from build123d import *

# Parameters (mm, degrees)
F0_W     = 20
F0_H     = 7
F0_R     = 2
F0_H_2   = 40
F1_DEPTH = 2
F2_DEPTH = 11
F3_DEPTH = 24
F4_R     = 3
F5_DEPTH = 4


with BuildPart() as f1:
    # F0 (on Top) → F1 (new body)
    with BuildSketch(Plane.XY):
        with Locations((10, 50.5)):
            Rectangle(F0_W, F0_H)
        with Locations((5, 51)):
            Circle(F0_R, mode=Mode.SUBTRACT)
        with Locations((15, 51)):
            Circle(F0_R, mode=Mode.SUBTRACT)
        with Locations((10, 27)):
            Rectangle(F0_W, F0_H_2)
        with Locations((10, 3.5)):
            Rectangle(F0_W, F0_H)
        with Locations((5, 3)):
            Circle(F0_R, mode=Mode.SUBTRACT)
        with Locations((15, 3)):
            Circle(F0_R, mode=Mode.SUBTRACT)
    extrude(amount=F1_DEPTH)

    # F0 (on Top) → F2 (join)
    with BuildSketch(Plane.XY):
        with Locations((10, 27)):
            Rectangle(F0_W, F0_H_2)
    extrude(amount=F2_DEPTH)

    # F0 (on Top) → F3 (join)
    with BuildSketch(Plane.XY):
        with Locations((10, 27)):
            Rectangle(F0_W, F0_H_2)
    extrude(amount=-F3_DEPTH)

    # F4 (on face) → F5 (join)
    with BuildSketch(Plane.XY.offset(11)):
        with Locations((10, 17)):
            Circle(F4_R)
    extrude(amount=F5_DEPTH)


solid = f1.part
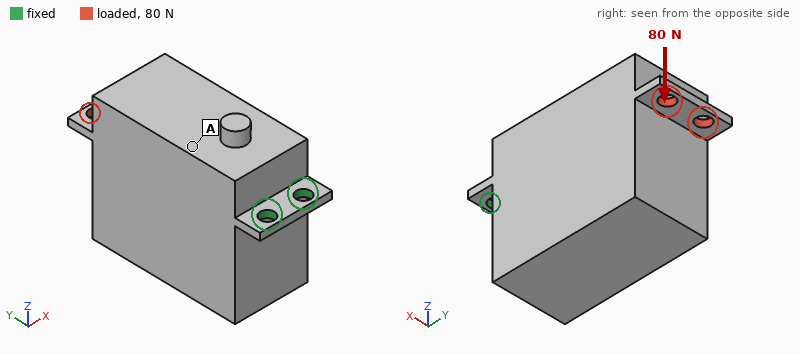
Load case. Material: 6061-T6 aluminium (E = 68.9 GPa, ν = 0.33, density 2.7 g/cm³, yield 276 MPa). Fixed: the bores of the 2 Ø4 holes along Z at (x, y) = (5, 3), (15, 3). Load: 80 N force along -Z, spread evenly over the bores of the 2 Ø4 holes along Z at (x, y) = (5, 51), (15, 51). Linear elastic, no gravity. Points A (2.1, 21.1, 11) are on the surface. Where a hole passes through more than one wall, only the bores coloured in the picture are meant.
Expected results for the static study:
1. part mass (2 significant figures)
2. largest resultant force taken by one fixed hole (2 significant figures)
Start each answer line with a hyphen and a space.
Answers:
- 77 g
- 40 N
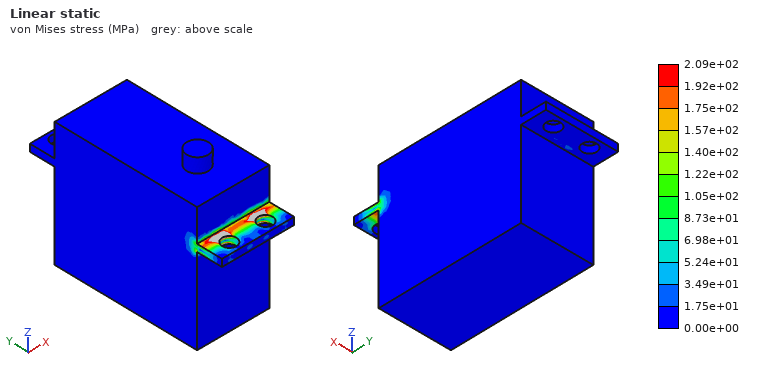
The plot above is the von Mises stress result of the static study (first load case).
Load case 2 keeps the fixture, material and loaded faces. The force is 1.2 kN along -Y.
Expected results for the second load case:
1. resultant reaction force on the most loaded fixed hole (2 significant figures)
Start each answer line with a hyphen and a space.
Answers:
- 600 N
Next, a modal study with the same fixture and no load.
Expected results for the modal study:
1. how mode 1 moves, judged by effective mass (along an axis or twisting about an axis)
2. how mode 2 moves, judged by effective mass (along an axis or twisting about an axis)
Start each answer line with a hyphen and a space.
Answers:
- along Z
- along X
